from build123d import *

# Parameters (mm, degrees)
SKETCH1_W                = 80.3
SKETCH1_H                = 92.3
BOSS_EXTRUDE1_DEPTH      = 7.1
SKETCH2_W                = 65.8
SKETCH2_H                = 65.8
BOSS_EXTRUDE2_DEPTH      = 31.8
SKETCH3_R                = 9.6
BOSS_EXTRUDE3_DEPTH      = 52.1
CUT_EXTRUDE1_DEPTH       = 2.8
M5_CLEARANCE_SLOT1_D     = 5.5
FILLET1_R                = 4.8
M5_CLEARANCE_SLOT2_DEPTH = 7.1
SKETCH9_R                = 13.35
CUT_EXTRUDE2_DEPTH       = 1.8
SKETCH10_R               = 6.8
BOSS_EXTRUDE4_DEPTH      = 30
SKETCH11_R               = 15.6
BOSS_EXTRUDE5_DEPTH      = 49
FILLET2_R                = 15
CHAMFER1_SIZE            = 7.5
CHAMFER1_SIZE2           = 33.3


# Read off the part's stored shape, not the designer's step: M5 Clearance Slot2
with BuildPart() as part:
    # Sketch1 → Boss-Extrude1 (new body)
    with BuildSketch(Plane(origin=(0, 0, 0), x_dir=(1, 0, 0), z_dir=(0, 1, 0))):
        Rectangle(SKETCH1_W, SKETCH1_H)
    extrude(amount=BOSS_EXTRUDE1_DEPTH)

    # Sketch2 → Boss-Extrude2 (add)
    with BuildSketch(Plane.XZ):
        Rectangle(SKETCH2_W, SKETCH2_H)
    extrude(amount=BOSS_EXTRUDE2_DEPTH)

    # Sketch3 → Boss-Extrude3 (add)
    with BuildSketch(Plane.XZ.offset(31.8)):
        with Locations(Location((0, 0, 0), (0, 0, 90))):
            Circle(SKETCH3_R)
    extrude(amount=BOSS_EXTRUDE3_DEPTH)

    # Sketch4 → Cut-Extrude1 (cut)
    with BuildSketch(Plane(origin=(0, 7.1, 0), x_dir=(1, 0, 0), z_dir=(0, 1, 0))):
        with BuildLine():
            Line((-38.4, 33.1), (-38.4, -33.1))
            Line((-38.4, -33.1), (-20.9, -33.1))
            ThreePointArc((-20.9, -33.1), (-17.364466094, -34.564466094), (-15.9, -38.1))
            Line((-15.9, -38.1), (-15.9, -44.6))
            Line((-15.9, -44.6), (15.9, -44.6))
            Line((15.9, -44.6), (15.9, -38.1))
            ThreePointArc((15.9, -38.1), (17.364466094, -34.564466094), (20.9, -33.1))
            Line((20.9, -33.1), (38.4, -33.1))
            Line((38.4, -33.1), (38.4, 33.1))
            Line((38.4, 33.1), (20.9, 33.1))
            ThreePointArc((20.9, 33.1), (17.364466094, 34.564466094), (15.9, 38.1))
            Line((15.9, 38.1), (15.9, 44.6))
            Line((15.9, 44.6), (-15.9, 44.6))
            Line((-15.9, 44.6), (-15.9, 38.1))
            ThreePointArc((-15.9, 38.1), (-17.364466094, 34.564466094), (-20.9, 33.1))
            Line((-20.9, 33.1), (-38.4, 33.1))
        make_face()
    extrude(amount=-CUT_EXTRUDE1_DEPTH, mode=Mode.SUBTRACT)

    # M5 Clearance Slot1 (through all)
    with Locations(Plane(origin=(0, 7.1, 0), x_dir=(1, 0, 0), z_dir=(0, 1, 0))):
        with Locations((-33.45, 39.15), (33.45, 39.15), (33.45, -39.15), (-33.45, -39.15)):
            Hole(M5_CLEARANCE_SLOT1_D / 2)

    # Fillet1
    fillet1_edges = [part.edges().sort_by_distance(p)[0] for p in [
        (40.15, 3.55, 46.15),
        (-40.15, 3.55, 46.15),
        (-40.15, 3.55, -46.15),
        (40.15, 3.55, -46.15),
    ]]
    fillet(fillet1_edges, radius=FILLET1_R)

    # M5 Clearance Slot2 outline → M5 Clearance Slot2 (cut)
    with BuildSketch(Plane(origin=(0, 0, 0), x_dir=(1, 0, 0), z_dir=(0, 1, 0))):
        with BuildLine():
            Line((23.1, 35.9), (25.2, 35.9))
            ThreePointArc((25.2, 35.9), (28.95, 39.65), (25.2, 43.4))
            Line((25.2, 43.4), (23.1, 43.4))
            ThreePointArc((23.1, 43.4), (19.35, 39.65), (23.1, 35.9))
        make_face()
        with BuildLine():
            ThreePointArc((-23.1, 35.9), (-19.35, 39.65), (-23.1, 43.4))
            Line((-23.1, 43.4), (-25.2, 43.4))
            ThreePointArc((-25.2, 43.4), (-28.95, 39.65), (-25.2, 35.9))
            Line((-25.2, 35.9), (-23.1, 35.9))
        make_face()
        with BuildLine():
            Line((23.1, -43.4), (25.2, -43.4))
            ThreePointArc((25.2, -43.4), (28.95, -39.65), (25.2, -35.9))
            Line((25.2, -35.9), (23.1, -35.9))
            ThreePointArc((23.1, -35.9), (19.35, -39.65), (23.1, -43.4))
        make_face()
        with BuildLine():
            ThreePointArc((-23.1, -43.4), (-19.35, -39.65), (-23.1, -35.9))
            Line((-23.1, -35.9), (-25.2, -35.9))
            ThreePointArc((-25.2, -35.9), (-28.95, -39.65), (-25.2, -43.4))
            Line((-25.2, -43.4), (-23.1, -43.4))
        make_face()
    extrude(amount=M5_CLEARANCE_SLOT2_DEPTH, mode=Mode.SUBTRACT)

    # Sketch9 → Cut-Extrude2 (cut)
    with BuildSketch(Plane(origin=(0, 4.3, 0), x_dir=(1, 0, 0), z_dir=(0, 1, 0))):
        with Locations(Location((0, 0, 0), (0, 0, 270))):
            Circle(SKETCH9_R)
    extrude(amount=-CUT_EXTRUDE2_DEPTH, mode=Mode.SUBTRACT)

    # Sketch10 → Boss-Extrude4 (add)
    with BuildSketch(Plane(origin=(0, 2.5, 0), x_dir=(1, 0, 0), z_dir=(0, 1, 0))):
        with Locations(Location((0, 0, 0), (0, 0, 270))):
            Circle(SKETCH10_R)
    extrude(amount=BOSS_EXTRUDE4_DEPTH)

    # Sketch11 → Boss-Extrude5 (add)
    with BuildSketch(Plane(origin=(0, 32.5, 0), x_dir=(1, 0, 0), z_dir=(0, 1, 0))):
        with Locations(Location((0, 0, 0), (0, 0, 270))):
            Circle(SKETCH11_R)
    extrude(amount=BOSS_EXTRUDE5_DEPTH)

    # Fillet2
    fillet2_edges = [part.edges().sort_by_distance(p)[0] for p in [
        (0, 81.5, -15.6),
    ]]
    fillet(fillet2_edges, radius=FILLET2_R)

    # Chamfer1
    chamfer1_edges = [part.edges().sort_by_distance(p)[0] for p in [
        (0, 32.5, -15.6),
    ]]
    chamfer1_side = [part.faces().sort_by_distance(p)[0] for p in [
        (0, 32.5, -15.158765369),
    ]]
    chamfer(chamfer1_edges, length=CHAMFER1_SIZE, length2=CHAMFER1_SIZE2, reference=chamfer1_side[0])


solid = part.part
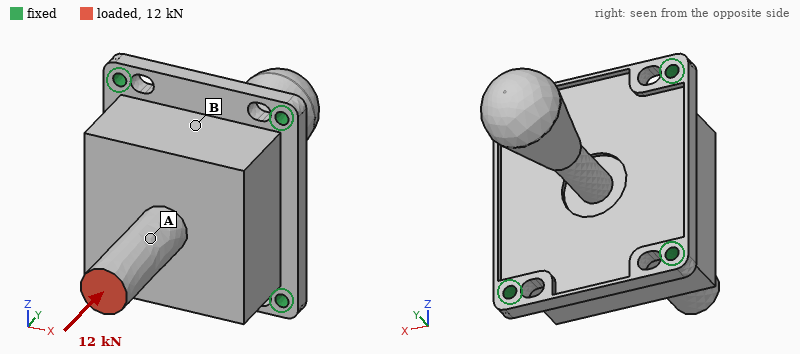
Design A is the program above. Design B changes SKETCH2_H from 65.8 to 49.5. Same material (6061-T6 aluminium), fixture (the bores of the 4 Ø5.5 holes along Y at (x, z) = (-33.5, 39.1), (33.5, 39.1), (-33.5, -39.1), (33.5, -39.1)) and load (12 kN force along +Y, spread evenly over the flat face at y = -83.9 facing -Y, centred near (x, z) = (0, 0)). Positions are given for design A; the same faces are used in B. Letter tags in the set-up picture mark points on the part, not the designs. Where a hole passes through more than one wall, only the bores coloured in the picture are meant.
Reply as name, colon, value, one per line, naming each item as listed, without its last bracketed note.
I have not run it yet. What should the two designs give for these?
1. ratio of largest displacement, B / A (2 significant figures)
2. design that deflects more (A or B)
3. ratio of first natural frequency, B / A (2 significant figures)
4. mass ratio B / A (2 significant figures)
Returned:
ratio of largest displacement, B / A: 2.0
design that deflects more: B
ratio of first natural frequency, B / A: 0.98
mass ratio B / A: 0.84
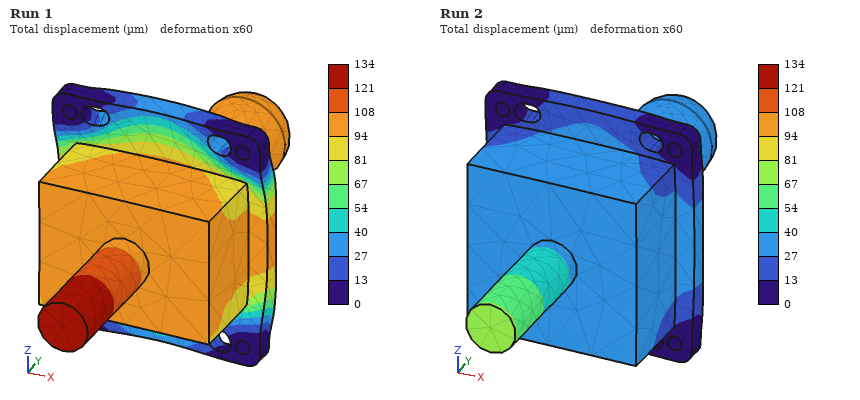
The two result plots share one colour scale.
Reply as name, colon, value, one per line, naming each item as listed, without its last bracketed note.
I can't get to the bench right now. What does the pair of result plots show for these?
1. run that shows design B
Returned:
run that shows design B: Run 1
